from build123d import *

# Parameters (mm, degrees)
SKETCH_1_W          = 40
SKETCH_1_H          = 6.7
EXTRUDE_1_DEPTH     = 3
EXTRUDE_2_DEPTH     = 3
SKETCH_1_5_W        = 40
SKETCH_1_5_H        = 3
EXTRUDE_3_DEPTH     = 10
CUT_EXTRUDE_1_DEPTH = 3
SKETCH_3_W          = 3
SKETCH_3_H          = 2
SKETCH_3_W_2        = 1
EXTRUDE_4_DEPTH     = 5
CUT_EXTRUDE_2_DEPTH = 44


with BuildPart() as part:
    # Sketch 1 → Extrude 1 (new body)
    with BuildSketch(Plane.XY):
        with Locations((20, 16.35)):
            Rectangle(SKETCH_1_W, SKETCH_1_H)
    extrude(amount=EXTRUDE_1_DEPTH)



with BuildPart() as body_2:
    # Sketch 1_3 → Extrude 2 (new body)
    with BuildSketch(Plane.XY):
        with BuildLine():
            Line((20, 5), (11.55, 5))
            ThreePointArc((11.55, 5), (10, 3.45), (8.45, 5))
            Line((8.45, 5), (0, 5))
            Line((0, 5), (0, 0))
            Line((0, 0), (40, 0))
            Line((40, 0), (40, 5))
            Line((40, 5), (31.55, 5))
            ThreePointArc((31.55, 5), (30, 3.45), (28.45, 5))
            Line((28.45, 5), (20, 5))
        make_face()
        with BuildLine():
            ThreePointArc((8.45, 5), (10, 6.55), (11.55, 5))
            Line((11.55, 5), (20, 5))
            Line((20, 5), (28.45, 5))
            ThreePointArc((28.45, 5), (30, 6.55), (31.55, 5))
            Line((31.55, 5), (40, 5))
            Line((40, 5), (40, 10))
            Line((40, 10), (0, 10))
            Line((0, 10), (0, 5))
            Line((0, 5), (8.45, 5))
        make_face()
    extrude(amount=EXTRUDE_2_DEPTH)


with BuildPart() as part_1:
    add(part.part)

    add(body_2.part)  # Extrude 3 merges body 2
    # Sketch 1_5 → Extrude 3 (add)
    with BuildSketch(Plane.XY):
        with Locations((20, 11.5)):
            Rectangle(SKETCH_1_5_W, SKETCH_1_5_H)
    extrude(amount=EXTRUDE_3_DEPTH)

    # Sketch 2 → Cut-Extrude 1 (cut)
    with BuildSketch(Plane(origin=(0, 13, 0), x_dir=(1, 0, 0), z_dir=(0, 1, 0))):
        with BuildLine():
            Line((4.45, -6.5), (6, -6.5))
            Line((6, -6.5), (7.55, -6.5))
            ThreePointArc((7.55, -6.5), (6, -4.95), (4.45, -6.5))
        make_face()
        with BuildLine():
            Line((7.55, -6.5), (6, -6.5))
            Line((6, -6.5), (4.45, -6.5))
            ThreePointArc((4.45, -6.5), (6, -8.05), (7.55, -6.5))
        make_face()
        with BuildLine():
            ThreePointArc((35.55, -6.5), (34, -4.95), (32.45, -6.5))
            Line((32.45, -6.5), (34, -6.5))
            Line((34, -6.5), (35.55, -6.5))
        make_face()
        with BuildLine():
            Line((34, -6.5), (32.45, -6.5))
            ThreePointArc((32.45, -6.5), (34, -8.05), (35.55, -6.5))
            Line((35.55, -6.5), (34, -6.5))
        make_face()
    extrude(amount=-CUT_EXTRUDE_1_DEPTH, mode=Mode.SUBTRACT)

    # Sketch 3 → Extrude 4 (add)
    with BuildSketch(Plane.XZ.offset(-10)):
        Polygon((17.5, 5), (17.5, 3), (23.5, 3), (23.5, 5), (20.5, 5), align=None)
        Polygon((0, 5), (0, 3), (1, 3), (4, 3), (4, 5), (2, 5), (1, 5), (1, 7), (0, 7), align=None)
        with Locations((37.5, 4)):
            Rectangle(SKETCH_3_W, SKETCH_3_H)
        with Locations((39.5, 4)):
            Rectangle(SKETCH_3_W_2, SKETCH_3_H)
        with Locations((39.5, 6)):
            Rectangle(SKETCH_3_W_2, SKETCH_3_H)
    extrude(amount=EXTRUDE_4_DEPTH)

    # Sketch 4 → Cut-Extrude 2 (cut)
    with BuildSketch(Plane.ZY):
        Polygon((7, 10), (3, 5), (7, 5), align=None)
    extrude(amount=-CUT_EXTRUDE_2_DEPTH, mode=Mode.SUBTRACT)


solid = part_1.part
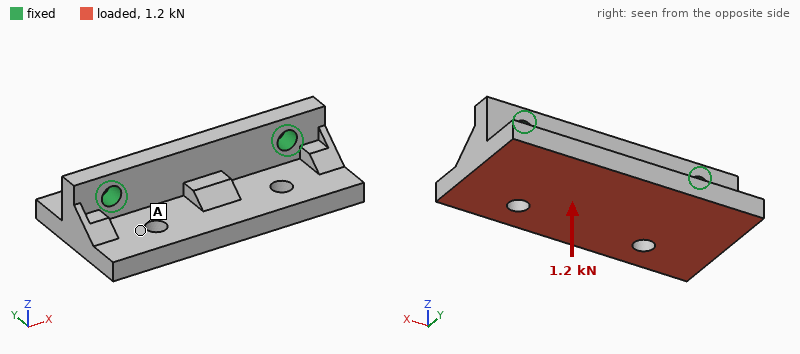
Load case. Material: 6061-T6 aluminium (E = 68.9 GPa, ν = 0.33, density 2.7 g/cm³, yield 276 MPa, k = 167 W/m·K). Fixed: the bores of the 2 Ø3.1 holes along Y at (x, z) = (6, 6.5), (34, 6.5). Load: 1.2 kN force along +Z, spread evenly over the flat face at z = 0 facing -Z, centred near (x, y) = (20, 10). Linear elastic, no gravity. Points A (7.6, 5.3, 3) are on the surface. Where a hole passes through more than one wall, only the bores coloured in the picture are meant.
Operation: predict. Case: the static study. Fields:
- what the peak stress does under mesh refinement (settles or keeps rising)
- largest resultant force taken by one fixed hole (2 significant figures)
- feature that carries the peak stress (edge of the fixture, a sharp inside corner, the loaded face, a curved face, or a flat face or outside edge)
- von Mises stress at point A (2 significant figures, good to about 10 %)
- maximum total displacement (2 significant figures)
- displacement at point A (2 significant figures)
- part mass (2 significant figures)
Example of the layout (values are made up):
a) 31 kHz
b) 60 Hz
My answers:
a) keeps rising
b) 630 N
c) edge of the fixture
d) 15 MPa
e) 36 µm
f) 14 µm
g) 8.7 g
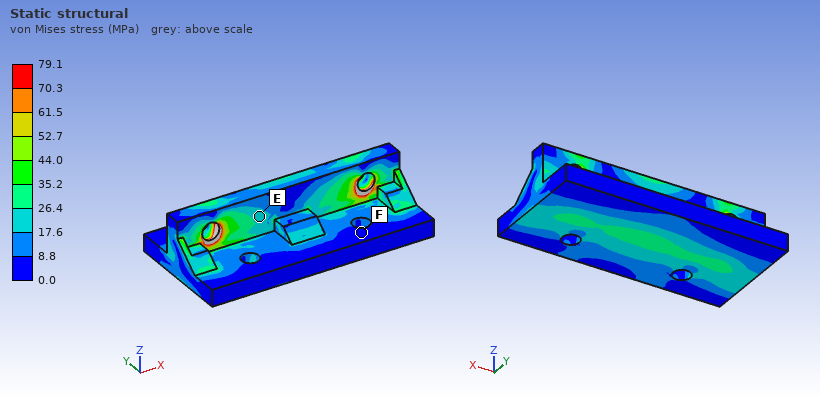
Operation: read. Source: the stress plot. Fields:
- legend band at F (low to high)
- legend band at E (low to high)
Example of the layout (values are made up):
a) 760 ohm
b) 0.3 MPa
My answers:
a) 0.0 to 8.8 MPa
b) 17.6 to 26.4 MPa
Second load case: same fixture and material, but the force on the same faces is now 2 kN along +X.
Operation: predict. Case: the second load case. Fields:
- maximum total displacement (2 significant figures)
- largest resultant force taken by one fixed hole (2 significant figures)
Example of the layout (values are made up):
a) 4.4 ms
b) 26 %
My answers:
a) 11 µm
b) 1.1 kN
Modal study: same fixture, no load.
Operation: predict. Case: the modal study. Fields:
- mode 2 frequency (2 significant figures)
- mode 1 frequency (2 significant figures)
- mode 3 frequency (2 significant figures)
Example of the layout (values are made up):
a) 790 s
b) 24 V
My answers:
a) 16 kHz
b) 9800 Hz
c) 22 kHz
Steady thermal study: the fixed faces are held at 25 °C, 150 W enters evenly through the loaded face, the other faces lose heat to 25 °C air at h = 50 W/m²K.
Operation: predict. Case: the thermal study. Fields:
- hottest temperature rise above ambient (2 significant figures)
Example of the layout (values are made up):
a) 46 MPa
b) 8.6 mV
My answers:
a) 76 K
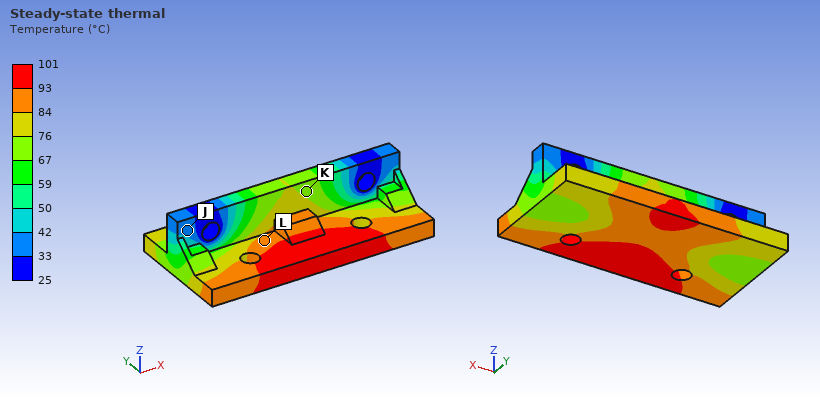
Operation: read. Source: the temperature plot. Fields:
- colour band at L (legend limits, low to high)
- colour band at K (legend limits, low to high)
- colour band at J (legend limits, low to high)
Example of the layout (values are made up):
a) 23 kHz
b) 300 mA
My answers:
a) 84 to 93 °C
b) 67 to 76 °C
c) 33 to 42 °C
